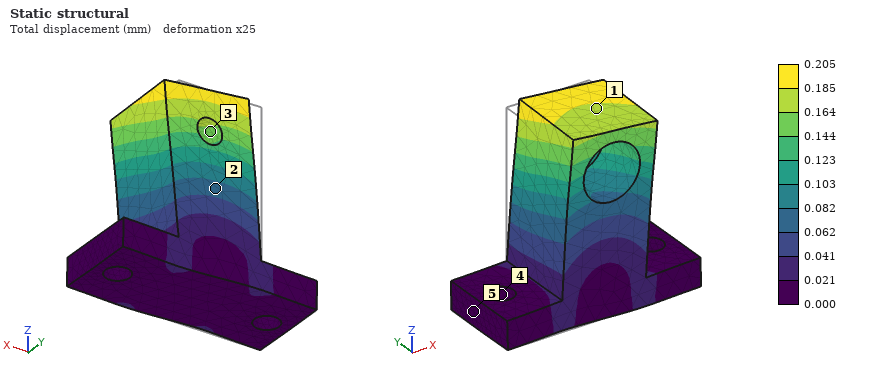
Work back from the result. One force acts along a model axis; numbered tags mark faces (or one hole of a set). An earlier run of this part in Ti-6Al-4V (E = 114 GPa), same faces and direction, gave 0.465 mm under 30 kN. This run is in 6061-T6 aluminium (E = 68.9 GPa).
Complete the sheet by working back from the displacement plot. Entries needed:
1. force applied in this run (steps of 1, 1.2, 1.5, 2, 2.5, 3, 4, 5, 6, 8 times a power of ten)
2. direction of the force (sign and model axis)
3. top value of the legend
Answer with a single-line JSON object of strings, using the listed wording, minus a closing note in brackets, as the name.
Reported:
{"force applied in this run": "8 kN", "direction of the force": "+X", "top value of the legend": "0.205 mm"}
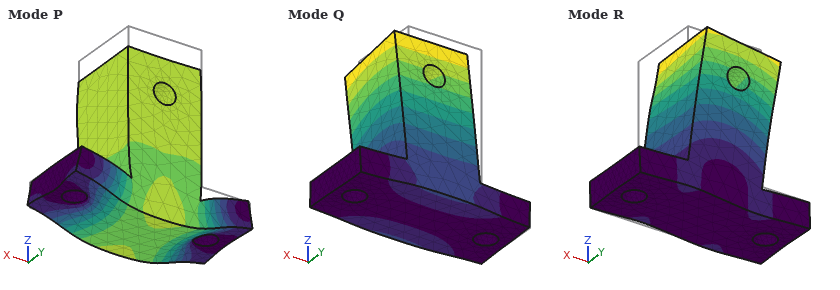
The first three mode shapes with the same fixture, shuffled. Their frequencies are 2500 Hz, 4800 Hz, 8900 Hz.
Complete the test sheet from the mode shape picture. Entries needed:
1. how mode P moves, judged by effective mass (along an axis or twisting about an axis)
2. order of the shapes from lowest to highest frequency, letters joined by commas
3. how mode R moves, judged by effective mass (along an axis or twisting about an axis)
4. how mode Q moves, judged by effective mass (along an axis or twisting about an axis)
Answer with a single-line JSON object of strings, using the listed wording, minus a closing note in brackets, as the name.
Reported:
{"how mode P moves, judged by effective mass": "along Z", "order of the shapes from lowest to highest frequency, letters joined by commas": "Q, R, P", "how mode R moves, judged by effective mass": "along X", "how mode Q moves, judged by effective mass": "along Y"}
